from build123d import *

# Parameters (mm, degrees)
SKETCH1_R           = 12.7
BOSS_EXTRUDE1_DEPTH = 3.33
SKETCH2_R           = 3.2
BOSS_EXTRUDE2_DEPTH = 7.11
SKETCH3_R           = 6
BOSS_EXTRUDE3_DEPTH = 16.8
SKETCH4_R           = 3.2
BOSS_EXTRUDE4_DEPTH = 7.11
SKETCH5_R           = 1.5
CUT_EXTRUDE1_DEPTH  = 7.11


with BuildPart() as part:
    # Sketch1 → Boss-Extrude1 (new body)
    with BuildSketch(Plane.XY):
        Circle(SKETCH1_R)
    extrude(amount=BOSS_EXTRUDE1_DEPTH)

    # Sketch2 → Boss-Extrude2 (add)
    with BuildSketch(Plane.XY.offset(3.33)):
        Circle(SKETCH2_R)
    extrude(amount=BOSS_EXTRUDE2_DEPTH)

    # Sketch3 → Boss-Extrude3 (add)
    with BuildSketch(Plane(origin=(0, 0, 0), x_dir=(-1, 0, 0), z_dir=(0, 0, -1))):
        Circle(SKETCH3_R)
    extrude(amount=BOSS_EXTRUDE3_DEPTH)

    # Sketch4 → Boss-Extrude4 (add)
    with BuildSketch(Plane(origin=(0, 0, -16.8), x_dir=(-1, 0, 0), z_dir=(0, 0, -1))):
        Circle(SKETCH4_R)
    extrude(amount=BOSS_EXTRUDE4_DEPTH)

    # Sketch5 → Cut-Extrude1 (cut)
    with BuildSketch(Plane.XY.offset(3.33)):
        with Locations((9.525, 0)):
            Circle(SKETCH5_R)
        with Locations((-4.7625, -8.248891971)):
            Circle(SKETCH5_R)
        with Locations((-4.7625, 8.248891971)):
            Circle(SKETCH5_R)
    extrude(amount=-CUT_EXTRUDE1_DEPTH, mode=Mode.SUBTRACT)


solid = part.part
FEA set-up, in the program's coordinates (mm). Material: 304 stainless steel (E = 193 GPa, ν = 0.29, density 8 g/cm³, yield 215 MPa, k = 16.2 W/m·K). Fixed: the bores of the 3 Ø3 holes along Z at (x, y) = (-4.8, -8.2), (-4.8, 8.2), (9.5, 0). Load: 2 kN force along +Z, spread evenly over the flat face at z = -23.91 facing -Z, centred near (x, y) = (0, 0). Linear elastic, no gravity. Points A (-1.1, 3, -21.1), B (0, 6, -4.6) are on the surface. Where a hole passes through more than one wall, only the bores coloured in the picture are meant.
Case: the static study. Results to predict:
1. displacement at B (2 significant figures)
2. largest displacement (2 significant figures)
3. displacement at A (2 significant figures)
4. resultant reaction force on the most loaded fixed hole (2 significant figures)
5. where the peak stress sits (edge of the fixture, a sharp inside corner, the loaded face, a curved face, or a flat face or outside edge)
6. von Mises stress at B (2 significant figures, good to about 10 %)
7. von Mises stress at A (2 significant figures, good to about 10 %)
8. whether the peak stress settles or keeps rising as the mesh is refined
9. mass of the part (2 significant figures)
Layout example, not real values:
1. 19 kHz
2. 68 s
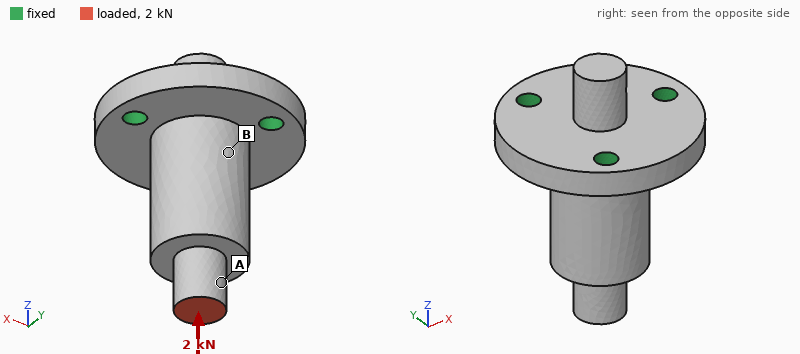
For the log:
1. 2.8 µm
2. 6.6 µm
3. 5.7 µm
4. 680 N
5. edge of the fixture
6. 17 MPa
7. 61 MPa
8. keeps rising
9. 32 g
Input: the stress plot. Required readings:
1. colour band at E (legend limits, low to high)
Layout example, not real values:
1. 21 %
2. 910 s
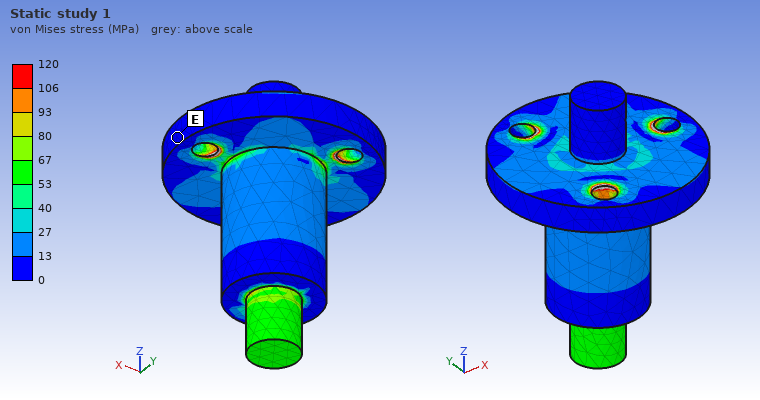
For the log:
1. 0 to 13 MPa
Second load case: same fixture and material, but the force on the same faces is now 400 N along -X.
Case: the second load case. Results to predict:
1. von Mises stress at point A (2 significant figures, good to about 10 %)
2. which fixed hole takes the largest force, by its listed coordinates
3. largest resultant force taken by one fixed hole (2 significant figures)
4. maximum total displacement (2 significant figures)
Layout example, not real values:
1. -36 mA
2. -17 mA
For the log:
1. 28 MPa
2. (9.5, 0)
3. 780 N
4. 27 µm
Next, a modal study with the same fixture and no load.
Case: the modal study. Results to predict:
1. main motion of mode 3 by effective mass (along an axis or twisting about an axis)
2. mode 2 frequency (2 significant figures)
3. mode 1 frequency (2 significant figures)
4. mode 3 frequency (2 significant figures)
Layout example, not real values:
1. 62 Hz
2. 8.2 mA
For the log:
1. along Z
2. 11 kHz
3. 11 kHz
4. 27 kHz
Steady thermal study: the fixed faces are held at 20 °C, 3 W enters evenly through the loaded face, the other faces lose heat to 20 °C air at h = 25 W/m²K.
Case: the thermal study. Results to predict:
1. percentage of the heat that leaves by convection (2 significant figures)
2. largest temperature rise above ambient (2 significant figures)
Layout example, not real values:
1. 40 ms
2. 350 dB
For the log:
1. 22 %
2. 75 K
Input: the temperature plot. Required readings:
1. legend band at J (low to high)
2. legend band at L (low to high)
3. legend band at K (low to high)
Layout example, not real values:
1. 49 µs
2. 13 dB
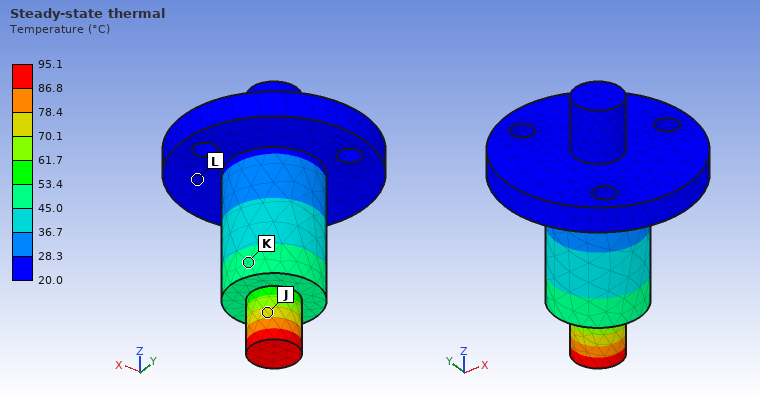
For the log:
1. 70.1 to 78.4 °C
2. 20.0 to 28.3 °C
3. 45.0 to 53.4 °C
